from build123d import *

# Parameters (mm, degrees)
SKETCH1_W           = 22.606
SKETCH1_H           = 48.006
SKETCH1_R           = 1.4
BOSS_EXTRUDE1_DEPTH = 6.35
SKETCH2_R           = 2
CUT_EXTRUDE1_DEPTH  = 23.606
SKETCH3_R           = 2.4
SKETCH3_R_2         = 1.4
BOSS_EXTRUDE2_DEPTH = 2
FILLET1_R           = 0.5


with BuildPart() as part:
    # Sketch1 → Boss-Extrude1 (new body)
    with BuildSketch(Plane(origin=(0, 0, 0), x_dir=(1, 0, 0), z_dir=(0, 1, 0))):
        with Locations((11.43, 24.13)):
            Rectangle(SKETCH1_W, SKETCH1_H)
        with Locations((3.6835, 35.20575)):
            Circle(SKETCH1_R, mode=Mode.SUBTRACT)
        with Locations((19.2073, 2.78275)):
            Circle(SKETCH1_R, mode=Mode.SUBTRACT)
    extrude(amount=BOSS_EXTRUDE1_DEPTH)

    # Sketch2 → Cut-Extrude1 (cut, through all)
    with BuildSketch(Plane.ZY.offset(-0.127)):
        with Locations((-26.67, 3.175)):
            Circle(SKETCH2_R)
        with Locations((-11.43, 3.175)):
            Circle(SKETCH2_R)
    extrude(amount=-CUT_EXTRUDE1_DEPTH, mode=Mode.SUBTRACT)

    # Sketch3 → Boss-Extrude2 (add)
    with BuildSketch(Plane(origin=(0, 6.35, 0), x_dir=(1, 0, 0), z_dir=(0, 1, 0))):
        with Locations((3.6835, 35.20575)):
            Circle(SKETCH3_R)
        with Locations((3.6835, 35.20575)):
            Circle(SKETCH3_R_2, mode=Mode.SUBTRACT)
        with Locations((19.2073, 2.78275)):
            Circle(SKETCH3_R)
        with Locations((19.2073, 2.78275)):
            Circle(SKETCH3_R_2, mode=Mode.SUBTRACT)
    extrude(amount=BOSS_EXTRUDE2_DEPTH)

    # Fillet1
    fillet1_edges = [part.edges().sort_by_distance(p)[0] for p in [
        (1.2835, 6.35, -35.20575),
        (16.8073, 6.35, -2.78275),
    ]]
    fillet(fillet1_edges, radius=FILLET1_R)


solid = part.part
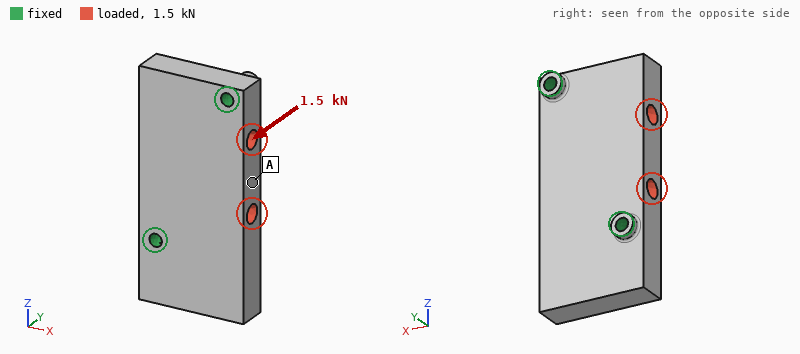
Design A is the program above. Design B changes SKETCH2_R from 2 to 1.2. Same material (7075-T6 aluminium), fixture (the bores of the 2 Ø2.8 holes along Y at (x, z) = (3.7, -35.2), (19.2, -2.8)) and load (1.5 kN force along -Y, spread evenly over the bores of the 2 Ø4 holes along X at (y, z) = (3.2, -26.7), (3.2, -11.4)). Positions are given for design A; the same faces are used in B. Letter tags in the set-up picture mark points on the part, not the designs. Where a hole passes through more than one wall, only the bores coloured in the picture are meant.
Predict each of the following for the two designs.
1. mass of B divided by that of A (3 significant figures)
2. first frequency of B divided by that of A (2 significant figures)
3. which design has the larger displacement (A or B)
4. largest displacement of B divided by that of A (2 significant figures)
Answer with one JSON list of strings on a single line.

["1.06", "1.0", "A", "0.87"]
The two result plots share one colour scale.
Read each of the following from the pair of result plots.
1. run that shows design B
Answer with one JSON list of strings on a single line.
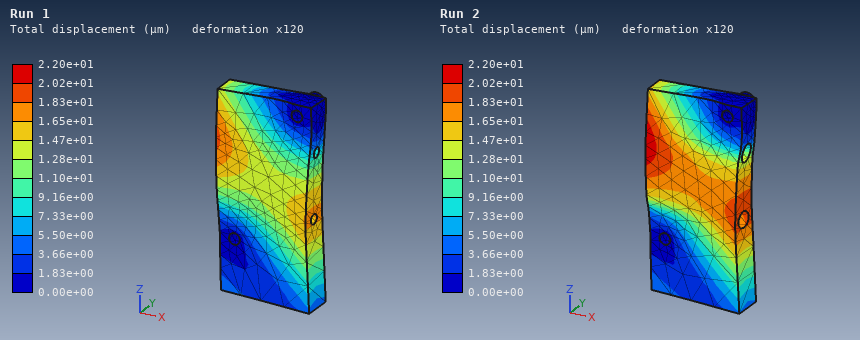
["Run 1"]
